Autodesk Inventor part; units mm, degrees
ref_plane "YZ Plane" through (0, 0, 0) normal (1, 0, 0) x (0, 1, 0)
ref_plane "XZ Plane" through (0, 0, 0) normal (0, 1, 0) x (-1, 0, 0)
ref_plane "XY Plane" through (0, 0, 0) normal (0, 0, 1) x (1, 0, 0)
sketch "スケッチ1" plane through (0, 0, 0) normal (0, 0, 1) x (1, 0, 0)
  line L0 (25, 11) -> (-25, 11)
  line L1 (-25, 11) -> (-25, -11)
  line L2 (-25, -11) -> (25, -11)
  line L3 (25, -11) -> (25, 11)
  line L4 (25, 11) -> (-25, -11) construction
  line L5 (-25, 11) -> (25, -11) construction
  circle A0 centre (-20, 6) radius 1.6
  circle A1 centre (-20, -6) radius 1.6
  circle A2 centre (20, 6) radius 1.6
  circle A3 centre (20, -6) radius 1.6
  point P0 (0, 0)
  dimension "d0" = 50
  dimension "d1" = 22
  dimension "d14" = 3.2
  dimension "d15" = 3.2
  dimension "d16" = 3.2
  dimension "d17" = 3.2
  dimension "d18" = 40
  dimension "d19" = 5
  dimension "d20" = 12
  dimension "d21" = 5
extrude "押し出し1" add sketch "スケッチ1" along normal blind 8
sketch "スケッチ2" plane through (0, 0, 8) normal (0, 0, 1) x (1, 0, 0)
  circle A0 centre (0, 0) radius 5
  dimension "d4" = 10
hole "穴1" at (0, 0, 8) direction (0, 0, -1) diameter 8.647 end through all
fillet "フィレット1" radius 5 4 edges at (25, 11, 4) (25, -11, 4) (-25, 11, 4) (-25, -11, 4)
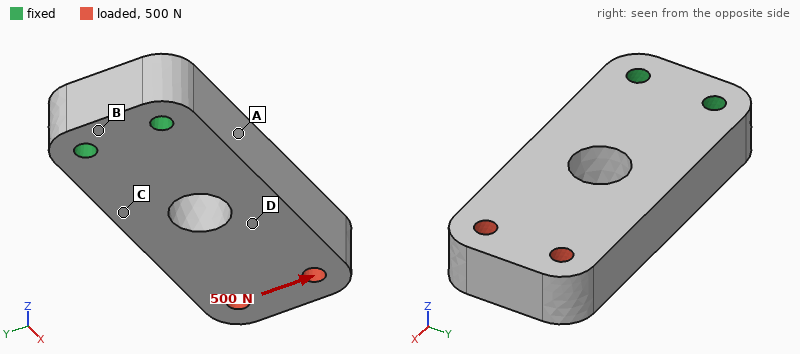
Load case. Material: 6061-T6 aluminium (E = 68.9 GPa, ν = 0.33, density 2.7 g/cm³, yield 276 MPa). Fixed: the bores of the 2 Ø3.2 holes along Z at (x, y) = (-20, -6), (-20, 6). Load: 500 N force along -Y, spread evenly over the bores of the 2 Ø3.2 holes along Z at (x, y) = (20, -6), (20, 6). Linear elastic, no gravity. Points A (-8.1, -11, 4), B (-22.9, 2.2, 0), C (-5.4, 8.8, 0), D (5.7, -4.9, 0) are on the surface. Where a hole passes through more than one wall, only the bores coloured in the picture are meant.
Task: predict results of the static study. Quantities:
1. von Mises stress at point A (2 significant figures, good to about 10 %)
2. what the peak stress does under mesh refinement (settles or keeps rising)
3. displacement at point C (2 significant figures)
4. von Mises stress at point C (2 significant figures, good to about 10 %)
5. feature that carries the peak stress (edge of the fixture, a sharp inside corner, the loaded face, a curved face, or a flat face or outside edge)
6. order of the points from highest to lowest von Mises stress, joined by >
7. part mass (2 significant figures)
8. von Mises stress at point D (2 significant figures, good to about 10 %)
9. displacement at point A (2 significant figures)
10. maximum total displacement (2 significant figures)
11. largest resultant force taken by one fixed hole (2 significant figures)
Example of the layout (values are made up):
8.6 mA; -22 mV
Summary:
26 MPa; keeps rising; 8.6 µm; 19 MPa; edge of the fixture; A > C > D > B; 21 g; 9.3 MPa; 7.8 µm; 37 µm; 1.4 kN
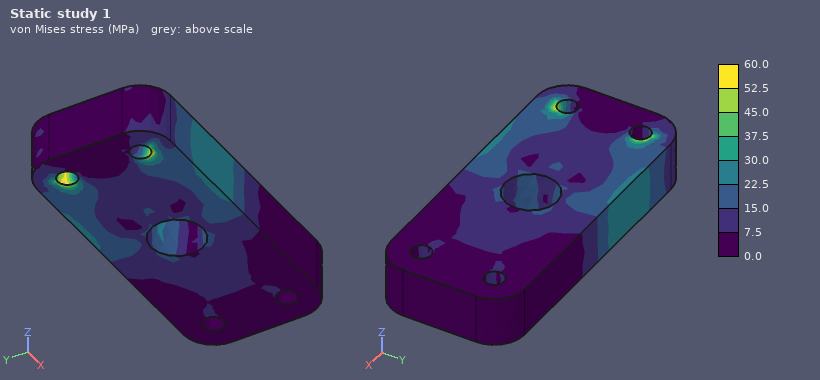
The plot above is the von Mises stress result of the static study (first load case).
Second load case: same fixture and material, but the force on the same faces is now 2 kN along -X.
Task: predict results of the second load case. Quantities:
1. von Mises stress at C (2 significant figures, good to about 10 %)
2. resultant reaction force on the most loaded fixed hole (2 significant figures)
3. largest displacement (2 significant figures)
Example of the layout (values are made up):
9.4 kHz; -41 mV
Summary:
17 MPa; 1.0 kN; 9.3 µm
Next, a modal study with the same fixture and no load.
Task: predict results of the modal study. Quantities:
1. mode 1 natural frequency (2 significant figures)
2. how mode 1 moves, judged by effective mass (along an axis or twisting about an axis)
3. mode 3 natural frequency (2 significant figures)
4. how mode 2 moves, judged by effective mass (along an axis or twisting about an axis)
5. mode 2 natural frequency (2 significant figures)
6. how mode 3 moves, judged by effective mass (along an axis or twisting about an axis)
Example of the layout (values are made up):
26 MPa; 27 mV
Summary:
3200 Hz; along Z; 11 kHz; along Y; 7200 Hz; twisting about X
